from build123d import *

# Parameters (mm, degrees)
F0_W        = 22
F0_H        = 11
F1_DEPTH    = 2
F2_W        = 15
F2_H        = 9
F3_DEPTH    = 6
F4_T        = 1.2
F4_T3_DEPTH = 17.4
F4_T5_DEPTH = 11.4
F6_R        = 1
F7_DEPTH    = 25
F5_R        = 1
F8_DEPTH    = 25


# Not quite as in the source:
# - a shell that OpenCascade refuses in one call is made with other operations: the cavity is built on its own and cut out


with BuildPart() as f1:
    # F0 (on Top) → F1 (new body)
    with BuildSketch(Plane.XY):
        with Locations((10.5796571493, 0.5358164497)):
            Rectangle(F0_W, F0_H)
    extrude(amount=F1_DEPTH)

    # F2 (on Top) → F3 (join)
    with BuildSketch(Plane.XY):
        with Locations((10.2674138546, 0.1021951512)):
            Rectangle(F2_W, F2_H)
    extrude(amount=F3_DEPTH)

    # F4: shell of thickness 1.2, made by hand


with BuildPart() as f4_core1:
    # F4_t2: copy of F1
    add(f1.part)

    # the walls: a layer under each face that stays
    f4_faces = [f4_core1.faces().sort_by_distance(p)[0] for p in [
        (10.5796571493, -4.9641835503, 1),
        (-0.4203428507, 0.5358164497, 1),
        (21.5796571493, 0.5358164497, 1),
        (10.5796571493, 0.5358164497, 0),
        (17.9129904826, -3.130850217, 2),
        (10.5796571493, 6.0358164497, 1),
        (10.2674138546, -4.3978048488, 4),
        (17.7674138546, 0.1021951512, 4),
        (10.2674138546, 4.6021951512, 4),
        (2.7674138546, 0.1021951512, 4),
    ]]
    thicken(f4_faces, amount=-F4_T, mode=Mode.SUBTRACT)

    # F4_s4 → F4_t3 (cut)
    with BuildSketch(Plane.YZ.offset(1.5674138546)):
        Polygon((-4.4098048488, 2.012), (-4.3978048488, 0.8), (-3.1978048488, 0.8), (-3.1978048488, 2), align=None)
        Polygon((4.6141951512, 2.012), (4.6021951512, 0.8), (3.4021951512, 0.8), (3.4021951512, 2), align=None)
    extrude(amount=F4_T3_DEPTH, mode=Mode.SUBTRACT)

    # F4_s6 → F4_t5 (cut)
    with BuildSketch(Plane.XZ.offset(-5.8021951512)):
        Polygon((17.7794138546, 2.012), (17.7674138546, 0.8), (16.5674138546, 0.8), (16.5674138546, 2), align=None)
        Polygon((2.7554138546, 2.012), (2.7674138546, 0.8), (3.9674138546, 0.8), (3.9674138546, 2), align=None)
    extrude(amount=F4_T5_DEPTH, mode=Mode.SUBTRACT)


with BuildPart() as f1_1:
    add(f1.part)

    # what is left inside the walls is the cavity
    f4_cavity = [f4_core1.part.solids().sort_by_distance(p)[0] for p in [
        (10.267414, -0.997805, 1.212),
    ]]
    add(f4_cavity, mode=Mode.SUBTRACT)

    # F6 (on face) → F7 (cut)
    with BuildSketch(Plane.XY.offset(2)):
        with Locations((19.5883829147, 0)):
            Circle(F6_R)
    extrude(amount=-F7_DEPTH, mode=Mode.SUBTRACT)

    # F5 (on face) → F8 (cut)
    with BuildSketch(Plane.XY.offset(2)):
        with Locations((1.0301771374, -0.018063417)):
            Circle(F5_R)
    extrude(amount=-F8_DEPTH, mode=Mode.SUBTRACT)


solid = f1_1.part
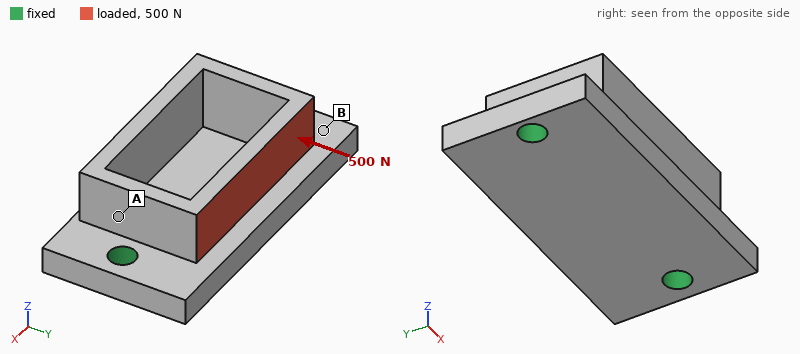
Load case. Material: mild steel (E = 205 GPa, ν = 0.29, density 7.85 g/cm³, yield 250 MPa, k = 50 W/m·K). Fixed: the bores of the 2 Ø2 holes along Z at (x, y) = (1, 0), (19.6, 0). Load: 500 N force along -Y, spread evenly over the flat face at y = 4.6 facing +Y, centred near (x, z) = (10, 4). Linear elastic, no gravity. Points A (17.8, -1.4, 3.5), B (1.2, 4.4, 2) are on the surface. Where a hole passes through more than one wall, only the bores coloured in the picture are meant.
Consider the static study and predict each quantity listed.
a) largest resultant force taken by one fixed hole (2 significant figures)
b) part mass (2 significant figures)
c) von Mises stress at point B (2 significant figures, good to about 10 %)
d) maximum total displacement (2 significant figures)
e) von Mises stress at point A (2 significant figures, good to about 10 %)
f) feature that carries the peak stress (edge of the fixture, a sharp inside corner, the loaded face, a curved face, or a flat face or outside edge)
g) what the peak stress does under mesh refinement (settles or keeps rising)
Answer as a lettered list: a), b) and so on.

a) 260 N
b) 4.8 g
c) 23 MPa
d) 25 µm
e) 60 MPa
f) edge of the fixture
g) keeps rising
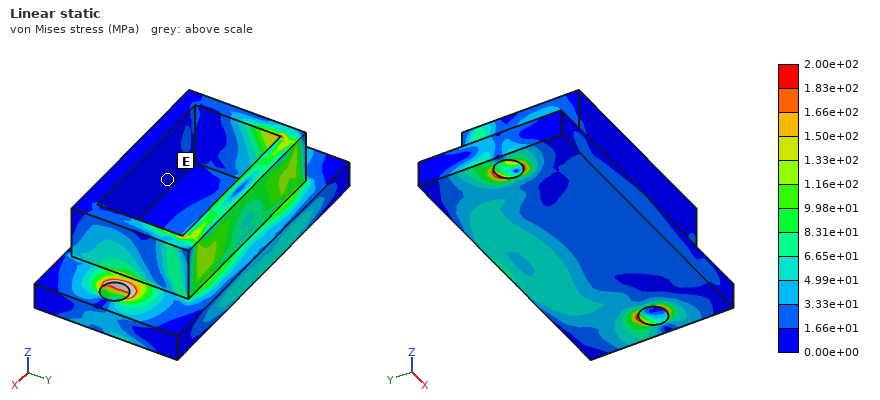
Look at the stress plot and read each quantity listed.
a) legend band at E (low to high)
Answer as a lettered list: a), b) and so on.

a) 0.00e+00 to 1.66e+01 MPa
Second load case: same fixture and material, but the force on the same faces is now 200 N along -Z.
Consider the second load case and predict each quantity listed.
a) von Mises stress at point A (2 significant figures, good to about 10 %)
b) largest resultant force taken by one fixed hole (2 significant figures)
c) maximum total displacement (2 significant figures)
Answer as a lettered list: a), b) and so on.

a) 21 MPa
b) 100 N
c) 7.4 µm
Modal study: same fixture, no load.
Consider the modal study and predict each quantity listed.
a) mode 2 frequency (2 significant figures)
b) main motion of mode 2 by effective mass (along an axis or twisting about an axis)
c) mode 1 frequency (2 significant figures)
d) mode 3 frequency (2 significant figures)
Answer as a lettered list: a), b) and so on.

a) 35 kHz
b) along Z
c) 23 kHz
d) 40 kHz
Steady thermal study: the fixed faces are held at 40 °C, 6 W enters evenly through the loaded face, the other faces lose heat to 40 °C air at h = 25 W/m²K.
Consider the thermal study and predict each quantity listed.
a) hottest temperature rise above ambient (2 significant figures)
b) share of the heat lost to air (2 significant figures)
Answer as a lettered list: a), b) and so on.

a) 37 K
b) 4.6 %
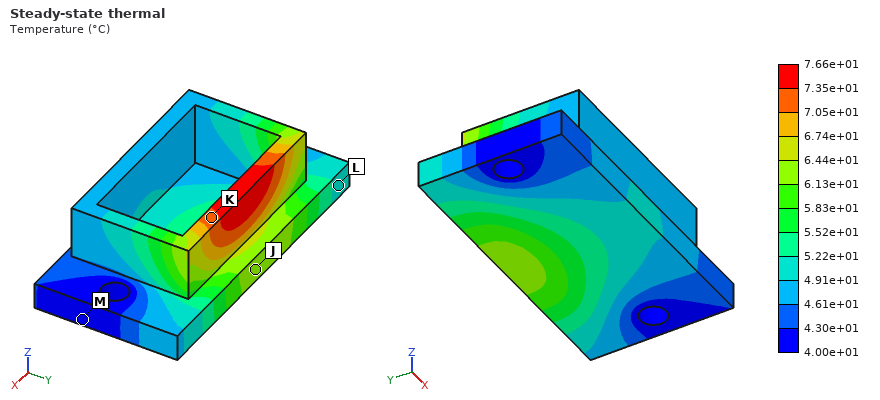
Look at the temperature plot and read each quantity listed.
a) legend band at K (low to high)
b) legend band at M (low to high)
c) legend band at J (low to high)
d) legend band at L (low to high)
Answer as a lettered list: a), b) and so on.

a) 7.05e+01 to 7.35e+01 °C
b) 4.00e+01 to 4.30e+01 °C
c) 6.13e+01 to 6.44e+01 °C
d) 4.91e+01 to 5.22e+01 °C
